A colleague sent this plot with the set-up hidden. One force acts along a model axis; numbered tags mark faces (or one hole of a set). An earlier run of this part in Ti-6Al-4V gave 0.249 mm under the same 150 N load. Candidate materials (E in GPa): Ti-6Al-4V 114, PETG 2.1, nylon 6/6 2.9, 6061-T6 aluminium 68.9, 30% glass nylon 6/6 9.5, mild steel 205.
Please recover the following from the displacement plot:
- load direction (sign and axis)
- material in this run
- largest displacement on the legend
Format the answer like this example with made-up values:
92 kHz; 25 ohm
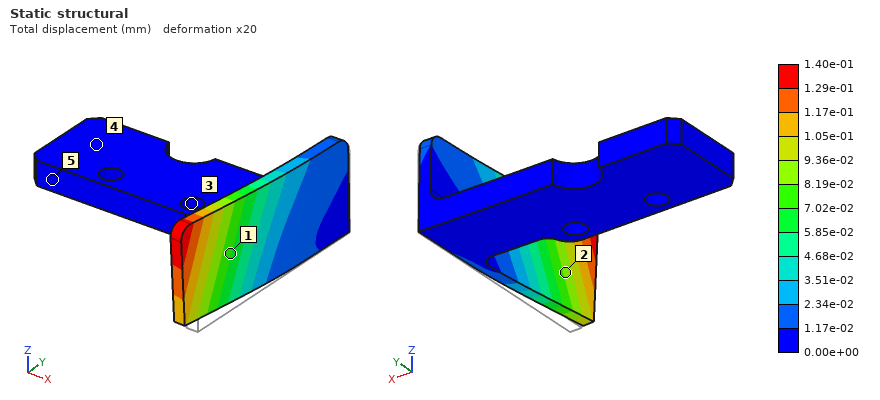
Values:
-X; mild steel; 1.40e-01 mm
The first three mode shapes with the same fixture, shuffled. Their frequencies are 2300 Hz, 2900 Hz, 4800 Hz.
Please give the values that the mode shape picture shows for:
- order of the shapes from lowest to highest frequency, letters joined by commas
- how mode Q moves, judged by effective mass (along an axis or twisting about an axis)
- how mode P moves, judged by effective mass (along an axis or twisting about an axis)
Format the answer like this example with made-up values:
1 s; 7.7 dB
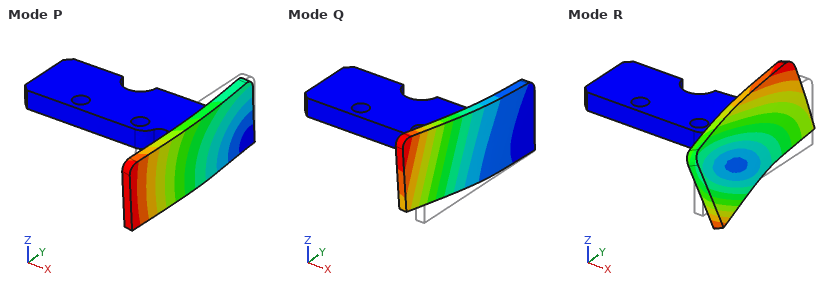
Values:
Q, P, R; along X; along Z
